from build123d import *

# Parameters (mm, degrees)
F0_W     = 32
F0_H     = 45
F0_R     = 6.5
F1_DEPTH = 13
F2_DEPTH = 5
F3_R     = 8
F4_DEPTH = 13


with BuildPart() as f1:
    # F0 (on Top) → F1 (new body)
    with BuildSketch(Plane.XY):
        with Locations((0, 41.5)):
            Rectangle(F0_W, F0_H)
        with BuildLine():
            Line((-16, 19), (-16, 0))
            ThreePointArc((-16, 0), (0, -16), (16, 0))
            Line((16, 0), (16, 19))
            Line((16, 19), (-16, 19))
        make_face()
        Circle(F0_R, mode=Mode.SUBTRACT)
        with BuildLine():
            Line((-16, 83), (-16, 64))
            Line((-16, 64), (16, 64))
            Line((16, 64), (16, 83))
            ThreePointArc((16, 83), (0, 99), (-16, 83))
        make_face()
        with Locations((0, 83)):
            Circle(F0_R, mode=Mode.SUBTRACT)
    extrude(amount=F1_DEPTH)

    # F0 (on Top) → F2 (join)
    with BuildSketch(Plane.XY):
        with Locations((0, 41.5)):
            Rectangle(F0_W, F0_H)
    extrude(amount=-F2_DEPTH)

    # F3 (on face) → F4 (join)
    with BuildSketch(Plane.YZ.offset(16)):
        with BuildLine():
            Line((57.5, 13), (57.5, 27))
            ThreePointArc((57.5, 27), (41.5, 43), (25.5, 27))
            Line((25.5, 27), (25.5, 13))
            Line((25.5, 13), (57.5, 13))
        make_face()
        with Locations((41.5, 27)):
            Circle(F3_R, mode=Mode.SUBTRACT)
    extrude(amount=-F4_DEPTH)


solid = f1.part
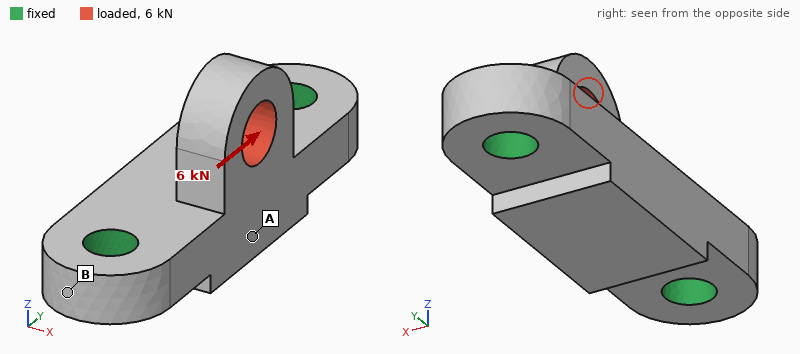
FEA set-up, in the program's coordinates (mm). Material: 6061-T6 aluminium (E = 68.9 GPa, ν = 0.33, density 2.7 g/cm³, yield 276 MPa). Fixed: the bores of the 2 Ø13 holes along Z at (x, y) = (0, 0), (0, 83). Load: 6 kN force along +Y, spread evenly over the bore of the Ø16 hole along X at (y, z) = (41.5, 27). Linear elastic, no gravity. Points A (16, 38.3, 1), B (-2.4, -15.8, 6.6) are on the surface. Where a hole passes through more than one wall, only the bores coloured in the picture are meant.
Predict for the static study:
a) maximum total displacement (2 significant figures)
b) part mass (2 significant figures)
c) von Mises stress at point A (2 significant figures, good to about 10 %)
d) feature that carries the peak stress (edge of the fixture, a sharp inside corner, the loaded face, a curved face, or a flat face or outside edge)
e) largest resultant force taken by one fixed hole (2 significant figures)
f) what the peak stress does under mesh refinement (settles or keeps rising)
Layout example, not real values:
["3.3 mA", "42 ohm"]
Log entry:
["68 µm", "150 g", "18 MPa", "a sharp inside corner", "3.7 kN", "keeps rising"]
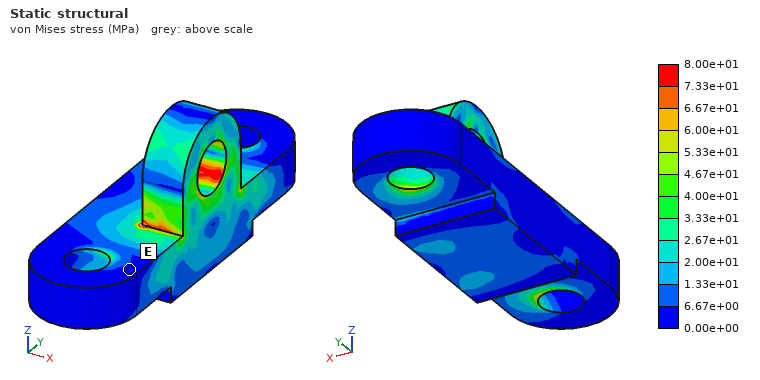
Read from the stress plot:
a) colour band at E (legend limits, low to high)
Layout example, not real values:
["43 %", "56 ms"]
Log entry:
["0.00e+00 to 6.67e+00 MPa"]
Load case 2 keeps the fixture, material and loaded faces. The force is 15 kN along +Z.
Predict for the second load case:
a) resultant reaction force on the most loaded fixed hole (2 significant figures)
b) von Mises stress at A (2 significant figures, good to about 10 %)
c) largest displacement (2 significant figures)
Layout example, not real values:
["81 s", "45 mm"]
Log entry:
["7.6 kN", "30 MPa", "0.16 mm"]
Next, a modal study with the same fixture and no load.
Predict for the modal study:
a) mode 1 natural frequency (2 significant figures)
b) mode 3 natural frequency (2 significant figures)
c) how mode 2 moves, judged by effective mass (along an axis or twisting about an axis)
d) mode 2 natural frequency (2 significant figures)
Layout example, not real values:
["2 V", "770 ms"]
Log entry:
["6100 Hz", "11 kHz", "along Z", "9200 Hz"]
